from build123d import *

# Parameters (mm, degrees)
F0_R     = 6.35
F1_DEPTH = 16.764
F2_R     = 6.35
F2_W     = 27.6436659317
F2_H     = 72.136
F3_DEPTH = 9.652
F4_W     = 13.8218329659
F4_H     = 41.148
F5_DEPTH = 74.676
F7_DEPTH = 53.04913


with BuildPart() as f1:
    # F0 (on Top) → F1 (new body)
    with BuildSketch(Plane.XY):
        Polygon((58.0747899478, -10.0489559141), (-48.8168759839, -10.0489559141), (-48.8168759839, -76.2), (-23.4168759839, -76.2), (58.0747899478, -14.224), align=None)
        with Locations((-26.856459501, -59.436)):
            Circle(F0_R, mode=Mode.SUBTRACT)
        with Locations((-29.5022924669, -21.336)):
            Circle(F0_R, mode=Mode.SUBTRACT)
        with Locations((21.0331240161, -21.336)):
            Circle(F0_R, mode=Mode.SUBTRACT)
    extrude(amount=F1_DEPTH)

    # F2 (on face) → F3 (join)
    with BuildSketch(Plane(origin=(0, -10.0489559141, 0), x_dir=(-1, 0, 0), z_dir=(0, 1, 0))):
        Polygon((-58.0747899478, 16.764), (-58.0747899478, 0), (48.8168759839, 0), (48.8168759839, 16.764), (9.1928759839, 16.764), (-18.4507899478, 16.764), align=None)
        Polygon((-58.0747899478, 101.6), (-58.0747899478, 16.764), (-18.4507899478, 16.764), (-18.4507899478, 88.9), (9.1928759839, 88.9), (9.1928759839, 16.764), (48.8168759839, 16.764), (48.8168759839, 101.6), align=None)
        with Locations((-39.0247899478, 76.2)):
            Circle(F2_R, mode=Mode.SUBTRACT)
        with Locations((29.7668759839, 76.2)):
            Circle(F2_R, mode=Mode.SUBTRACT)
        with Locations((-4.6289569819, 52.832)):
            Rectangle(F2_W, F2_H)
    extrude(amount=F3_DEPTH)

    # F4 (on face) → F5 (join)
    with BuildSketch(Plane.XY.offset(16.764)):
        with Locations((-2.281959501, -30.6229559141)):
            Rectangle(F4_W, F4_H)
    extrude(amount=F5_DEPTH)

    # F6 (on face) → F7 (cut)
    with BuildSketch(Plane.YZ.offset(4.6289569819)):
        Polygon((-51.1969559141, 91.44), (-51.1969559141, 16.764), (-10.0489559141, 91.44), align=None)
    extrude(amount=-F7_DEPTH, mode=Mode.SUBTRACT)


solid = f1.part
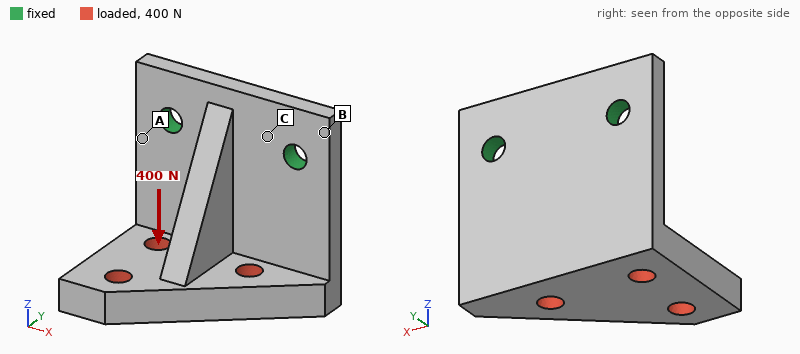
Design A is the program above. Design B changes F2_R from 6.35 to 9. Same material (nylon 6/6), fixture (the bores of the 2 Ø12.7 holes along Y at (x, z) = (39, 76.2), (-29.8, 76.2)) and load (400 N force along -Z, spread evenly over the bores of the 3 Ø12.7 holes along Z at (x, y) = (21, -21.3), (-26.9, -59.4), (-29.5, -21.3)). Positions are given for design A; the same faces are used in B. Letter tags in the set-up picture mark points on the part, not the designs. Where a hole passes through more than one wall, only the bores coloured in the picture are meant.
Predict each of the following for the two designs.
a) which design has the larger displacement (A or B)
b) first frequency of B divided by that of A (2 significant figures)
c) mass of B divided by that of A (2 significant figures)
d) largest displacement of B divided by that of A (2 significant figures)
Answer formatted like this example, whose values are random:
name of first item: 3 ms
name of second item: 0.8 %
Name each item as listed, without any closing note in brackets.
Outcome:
which design has the larger displacement: A
first frequency of B divided by that of A: 1.1
mass of B divided by that of A: 0.99
largest displacement of B divided by that of A: 0.84
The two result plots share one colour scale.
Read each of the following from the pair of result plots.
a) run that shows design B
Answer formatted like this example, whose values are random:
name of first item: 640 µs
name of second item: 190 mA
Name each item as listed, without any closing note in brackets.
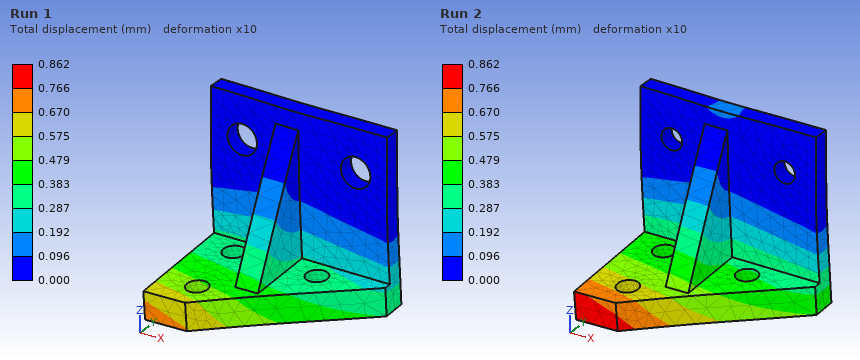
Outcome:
run that shows design B: Run 1
